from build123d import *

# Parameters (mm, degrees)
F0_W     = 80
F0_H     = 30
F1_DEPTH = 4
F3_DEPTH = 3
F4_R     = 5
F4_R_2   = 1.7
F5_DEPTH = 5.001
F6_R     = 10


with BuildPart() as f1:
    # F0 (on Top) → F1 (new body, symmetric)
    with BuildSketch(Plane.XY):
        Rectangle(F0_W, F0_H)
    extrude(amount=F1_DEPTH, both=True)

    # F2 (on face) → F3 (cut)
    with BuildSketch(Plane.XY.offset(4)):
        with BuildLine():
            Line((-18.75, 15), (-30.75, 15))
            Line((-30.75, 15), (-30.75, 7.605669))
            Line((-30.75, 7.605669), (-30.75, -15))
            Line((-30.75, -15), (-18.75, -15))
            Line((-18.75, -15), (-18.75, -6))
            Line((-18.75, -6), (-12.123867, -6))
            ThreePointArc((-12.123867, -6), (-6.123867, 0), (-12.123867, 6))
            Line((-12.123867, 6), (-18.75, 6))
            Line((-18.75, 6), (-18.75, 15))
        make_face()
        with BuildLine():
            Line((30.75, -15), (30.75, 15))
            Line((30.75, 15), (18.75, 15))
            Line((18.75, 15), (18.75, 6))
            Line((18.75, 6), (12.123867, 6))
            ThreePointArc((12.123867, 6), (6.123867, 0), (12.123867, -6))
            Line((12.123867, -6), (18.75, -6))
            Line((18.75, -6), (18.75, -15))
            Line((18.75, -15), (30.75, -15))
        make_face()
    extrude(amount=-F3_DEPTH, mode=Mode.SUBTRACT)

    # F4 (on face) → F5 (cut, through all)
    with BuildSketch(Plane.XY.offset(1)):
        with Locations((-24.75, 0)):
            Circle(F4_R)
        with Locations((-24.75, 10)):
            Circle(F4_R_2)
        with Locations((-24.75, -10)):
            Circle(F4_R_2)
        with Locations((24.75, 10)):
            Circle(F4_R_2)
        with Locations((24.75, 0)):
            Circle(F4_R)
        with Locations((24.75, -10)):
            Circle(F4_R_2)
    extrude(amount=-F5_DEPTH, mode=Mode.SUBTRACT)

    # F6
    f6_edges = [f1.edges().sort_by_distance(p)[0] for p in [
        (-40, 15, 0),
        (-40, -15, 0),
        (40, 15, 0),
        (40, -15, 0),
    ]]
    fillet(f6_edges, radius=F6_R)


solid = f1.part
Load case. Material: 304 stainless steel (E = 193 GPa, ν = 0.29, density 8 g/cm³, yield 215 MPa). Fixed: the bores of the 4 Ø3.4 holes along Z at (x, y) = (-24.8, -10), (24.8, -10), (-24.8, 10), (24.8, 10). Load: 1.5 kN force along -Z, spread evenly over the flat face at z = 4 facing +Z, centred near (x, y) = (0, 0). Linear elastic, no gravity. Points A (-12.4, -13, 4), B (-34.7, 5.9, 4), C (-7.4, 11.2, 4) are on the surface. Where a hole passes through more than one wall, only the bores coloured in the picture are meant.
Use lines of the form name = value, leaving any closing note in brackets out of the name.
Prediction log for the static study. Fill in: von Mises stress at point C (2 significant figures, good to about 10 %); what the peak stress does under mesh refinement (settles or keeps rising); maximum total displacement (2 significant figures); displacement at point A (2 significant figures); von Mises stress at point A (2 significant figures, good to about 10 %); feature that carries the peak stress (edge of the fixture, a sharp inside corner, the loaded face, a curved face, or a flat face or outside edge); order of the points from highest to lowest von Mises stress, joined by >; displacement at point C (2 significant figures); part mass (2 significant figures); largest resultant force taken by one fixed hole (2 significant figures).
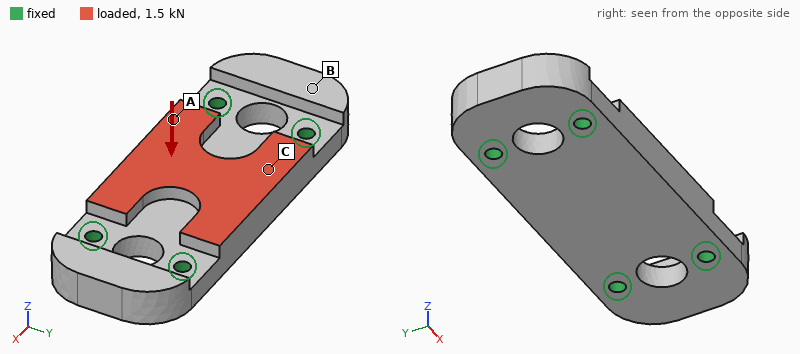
von Mises stress at point C = 22 MPa
what the peak stress does under mesh refinement = keeps rising
maximum total displacement = 6.9 µm
displacement at point A = 4.6 µm
von Mises stress at point A = 14 MPa
feature that carries the peak stress = edge of the fixture
order of the points from highest to lowest von Mises stress, joined by > = C > A > B
displacement at point C = 5.8 µm
part mass = 120 g
largest resultant force taken by one fixed hole = 470 N
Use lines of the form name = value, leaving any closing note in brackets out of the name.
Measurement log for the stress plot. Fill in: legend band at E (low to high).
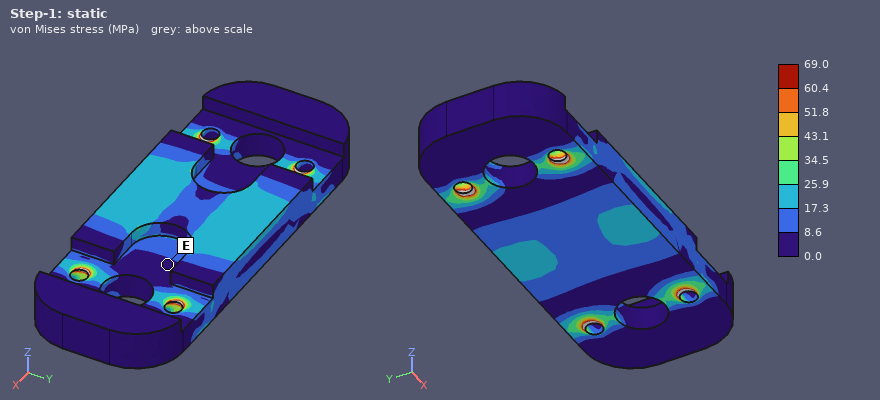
legend band at E = 0.0 to 8.6 MPa
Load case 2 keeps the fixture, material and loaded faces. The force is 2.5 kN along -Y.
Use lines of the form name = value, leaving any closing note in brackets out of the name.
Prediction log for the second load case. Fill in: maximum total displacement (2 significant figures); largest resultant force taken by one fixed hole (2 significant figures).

maximum total displacement = 8.1 µm
largest resultant force taken by one fixed hole = 900 N
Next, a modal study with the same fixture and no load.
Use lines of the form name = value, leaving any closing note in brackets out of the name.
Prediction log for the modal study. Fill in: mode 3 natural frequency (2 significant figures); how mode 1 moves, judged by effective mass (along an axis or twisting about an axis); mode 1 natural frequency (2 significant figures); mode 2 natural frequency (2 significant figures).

mode 3 natural frequency = 13 kHz
how mode 1 moves, judged by effective mass = along Z
mode 1 natural frequency = 10 kHz
mode 2 natural frequency = 12 kHz
